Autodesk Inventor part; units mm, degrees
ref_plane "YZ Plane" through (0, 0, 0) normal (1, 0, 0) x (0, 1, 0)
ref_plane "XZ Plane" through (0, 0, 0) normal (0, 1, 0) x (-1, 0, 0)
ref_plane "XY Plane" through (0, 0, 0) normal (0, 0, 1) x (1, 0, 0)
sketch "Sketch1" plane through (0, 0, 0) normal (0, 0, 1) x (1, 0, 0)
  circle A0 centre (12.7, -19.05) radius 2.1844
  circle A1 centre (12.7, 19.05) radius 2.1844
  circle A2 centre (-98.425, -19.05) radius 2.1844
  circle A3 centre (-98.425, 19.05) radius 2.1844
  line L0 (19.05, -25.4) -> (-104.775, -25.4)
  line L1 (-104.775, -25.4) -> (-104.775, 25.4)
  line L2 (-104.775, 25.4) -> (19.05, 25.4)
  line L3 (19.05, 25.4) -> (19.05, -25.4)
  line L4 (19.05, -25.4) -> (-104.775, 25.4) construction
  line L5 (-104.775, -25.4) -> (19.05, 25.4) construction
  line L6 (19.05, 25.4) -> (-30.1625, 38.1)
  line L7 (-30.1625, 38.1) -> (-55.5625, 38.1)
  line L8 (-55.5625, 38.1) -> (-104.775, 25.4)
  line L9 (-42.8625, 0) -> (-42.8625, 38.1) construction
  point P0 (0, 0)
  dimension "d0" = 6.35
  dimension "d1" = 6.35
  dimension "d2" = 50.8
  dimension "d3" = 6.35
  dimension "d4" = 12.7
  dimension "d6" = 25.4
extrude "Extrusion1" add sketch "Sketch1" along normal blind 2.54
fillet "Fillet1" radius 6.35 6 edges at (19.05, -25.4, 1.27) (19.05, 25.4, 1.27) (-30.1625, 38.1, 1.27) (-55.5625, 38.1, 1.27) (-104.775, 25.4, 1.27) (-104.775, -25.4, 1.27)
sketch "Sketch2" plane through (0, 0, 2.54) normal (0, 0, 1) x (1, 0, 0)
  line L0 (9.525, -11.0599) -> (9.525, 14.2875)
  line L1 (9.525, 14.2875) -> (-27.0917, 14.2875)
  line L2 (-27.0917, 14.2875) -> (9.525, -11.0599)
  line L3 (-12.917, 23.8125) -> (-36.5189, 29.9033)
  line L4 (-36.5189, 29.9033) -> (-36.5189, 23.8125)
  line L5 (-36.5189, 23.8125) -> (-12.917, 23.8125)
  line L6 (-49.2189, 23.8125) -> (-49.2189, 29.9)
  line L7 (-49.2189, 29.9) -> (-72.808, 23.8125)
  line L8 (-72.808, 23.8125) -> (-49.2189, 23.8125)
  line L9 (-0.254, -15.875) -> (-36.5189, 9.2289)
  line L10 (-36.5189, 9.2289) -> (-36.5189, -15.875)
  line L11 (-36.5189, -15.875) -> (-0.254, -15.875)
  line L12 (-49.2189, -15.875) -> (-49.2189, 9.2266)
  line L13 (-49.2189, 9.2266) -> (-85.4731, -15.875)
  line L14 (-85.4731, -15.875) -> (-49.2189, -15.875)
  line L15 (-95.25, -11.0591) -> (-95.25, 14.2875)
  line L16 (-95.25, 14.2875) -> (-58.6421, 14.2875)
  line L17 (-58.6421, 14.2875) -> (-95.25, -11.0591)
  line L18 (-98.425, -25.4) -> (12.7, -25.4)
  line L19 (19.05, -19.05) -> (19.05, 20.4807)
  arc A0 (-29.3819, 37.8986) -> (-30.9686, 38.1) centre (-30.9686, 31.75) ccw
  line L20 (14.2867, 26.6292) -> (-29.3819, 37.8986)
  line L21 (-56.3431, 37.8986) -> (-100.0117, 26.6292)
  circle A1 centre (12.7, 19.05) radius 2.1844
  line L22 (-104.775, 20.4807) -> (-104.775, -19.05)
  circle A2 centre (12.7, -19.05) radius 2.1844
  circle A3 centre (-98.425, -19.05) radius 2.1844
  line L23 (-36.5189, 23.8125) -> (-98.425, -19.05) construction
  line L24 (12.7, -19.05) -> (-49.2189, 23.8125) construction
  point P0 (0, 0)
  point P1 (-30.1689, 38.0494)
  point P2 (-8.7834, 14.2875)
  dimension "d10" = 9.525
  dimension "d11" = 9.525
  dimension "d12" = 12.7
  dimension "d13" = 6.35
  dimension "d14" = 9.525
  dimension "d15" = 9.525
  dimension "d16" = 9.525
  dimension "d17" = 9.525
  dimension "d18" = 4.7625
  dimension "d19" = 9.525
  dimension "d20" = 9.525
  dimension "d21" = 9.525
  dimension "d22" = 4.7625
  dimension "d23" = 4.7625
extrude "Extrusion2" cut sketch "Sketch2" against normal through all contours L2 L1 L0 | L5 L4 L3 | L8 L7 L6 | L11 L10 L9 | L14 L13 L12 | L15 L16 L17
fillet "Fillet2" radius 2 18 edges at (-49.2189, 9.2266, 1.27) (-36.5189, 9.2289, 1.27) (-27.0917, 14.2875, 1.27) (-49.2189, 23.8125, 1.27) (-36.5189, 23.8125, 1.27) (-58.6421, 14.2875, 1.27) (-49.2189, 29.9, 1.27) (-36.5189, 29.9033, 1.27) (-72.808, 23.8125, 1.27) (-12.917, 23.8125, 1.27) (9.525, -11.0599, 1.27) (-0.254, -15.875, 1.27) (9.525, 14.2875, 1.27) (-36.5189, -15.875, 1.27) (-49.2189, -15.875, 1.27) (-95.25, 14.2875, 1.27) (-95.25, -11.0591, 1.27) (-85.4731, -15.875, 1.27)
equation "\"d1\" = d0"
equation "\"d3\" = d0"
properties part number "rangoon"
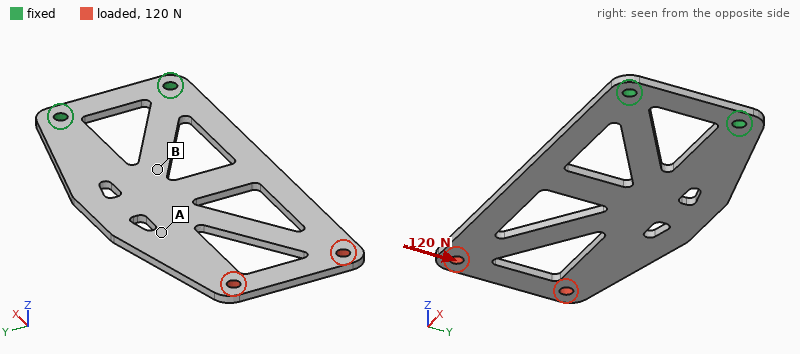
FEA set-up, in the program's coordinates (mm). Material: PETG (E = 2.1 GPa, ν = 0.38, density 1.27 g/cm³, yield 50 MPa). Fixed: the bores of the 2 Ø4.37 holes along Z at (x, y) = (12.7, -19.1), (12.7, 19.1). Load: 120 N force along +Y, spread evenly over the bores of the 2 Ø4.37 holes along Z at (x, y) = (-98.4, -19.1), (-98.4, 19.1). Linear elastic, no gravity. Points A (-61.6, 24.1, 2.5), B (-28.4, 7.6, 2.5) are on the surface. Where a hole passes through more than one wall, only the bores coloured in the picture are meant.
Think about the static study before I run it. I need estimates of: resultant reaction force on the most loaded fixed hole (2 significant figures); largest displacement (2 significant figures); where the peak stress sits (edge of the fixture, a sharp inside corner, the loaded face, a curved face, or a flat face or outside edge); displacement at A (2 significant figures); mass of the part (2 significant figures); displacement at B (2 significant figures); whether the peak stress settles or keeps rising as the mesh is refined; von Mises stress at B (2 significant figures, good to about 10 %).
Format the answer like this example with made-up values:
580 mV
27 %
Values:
340 N
1.6 mm
edge of the fixture
0.91 mm
17 g
0.43 mm
keeps rising
7.0 MPa
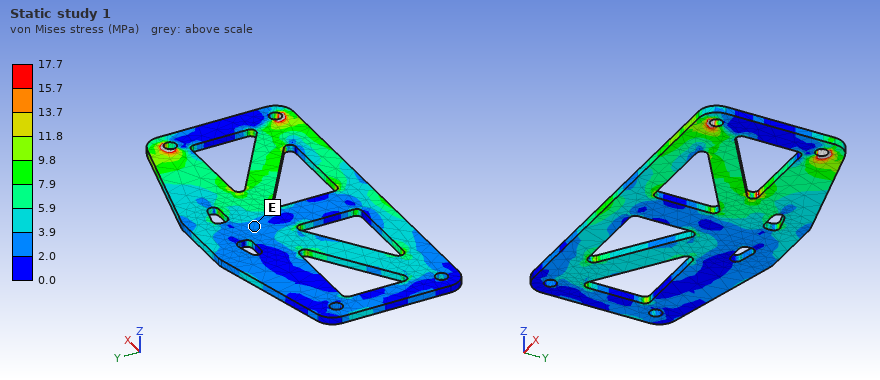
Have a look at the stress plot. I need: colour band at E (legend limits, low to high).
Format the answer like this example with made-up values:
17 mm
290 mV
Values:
2.0 to 3.9 MPa
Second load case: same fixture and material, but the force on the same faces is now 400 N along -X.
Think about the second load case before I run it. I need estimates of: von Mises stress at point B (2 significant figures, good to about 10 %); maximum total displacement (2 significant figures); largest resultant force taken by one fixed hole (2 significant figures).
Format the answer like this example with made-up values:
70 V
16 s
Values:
2.8 MPa
0.44 mm
210 N
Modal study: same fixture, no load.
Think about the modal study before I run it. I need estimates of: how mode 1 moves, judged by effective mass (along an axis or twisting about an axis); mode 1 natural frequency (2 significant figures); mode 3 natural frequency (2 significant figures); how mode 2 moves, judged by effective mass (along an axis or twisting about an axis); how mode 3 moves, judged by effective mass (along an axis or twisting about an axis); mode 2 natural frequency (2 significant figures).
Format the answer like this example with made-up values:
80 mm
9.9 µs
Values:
along Z
36 Hz
220 Hz
twisting about X
along Z
140 Hz
